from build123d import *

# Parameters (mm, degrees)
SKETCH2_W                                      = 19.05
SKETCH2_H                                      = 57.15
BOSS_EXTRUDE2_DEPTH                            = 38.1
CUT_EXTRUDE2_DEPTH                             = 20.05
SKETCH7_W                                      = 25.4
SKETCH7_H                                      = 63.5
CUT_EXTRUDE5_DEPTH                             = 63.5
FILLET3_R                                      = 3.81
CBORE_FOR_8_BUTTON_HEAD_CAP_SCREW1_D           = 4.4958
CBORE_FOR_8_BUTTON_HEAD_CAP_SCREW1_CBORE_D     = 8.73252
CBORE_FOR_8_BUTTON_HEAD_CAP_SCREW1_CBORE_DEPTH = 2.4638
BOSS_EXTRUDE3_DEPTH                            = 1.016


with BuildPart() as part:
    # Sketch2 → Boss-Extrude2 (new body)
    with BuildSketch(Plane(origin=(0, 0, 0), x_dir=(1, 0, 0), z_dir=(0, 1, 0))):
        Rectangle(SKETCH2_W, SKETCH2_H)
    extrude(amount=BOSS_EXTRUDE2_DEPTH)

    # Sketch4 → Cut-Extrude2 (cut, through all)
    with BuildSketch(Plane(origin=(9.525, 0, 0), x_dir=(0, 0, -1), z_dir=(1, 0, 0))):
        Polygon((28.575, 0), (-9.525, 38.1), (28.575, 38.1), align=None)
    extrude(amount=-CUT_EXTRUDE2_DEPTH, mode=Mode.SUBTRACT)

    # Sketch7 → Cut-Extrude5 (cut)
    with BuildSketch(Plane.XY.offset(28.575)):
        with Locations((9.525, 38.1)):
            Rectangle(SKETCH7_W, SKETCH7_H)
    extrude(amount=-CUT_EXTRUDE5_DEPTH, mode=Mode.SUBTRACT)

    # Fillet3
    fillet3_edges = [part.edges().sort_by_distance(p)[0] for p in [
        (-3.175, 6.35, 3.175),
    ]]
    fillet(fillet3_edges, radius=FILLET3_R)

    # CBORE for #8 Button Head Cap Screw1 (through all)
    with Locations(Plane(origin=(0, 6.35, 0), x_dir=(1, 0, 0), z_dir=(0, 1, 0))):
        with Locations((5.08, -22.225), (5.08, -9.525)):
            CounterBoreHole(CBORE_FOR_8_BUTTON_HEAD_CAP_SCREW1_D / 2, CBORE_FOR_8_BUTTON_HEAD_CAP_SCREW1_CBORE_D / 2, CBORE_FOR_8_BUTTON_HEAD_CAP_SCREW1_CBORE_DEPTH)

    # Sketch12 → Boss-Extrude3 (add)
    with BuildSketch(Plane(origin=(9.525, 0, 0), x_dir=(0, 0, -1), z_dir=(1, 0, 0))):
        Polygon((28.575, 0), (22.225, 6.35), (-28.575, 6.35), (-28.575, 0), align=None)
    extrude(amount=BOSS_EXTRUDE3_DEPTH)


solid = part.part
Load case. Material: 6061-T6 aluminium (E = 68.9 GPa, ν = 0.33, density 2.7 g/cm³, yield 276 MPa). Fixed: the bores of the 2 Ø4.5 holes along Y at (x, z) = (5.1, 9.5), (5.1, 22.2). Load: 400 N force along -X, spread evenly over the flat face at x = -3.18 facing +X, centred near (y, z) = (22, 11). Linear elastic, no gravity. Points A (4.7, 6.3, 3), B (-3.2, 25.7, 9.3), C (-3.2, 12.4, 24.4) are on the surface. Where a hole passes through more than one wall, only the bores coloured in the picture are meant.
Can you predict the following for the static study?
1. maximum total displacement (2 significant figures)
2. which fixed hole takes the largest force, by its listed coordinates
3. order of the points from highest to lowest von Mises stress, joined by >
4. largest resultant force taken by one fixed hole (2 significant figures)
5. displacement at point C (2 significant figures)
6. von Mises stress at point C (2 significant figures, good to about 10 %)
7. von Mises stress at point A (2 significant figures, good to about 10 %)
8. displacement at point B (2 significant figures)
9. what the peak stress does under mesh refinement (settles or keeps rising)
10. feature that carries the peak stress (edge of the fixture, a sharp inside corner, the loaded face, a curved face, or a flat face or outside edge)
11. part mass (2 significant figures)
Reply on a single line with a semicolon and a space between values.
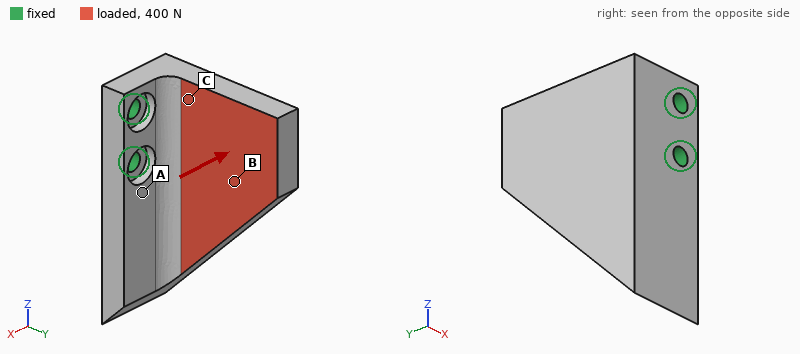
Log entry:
0.12 mm; (5.1, 9.5); A > C > B; 310 N; 0.028 mm; 17 MPa; 35 MPa; 0.073 mm; keeps rising; edge of the fixture; 37 g
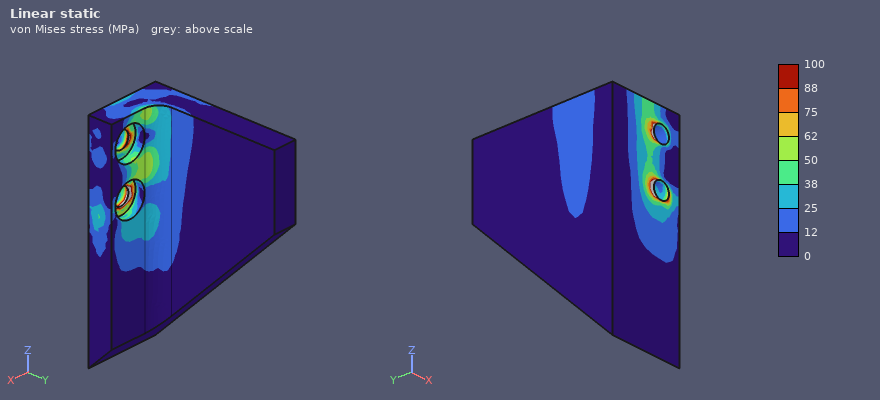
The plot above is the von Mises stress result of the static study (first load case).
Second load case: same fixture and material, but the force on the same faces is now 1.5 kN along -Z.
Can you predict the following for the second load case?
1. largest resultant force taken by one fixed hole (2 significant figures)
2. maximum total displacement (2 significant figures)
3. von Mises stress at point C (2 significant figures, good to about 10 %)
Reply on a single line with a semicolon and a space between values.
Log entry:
2.1 kN; 0.15 mm; 51 MPa
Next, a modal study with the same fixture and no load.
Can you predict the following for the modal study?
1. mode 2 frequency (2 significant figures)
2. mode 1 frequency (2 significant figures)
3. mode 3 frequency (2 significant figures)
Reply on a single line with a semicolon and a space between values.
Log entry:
3800 Hz; 2700 Hz; 6700 Hz
